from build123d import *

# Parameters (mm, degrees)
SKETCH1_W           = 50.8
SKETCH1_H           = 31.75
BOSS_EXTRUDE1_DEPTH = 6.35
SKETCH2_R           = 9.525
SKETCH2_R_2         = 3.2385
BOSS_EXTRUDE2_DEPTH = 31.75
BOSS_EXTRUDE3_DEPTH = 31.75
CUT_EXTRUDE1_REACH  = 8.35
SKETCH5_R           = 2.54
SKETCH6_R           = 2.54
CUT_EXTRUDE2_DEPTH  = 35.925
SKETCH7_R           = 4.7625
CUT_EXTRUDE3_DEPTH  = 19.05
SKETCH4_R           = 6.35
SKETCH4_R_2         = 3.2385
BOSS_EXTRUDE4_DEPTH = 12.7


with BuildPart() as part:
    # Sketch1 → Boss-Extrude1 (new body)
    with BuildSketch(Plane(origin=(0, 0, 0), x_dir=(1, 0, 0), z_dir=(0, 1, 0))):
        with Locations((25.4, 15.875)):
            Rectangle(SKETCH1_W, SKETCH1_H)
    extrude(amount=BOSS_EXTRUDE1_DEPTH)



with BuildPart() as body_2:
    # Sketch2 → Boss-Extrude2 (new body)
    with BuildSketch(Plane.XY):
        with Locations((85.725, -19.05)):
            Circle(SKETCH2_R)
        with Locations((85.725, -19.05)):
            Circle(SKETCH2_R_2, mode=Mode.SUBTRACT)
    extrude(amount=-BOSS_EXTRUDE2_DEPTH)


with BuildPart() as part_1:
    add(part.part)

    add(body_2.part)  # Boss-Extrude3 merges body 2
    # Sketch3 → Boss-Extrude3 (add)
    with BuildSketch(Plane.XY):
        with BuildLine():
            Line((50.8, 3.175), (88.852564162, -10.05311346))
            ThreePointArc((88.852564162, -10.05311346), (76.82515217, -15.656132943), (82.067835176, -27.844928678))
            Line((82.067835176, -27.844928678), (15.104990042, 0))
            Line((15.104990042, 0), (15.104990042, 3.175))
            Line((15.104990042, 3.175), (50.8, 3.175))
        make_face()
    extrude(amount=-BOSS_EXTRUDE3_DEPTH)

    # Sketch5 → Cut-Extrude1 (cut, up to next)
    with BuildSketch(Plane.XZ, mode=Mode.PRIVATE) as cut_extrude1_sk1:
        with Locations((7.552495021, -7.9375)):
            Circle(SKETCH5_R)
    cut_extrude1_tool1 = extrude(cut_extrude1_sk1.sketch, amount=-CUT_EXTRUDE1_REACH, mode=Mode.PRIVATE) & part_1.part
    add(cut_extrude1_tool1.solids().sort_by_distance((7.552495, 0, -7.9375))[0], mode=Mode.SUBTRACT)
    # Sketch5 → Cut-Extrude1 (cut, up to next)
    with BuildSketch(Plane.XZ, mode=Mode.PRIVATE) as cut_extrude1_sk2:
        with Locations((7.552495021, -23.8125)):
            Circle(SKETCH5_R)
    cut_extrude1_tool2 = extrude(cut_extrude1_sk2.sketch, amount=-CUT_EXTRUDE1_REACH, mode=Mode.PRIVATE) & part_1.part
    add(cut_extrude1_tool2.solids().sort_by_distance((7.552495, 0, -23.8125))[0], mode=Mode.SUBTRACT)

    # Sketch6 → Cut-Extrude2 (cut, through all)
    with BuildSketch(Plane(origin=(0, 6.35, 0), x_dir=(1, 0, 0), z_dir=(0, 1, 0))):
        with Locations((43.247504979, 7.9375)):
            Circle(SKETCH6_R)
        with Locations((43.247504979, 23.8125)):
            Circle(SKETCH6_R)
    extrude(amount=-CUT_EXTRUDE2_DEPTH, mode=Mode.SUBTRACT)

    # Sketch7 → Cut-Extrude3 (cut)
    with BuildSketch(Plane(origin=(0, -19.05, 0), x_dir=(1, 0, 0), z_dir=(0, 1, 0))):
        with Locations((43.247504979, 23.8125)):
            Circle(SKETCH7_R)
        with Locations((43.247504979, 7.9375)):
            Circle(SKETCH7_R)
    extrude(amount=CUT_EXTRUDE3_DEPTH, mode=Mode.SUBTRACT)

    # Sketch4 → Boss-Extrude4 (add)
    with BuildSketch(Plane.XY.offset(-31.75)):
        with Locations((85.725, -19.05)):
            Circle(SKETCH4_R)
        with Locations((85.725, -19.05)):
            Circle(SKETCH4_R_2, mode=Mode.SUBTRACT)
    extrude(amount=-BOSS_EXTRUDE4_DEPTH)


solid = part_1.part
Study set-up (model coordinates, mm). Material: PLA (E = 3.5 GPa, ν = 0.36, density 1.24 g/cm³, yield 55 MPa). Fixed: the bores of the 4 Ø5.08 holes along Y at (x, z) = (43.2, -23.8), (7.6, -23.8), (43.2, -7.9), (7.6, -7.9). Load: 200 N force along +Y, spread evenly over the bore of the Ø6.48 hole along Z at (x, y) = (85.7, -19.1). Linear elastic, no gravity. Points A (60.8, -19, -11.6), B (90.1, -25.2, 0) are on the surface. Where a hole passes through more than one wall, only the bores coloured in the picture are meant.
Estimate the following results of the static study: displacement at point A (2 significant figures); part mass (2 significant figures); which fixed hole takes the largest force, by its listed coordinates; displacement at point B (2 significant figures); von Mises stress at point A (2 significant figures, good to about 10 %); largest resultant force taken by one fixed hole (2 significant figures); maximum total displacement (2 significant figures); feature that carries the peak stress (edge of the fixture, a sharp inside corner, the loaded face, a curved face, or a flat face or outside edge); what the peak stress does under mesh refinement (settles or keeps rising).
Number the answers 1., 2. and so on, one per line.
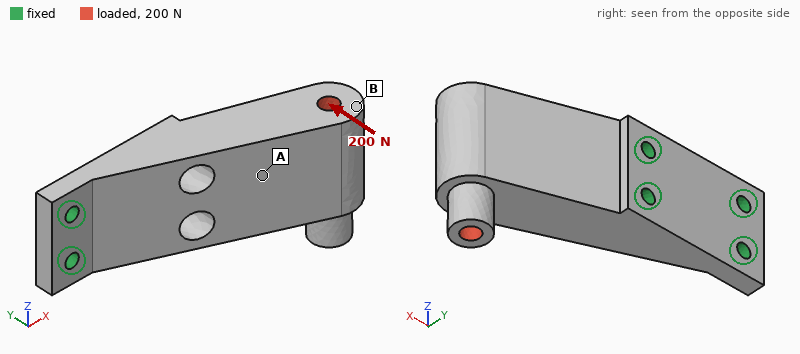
1. 0.14 mm
2. 53 g
3. (43.2, -23.8)
4. 0.32 mm
5. 2.6 MPa
6. 280 N
7. 0.39 mm
8. edge of the fixture
9. keeps rising
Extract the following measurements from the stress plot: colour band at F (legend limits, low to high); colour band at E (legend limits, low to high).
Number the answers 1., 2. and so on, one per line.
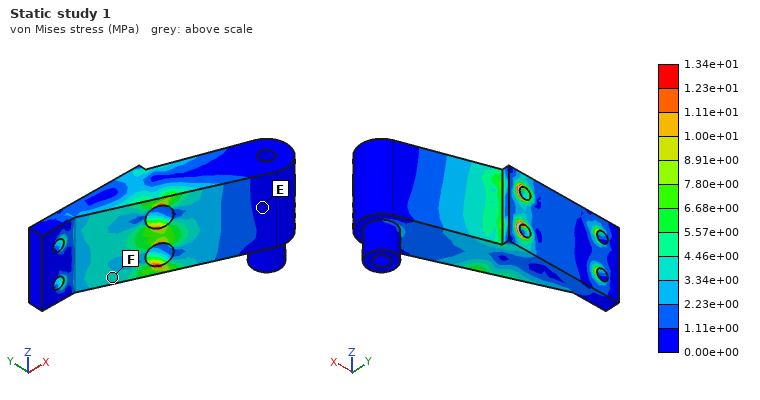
1. 3.34e+00 to 4.46e+00 MPa
2. 0.00e+00 to 1.11e+00 MPa
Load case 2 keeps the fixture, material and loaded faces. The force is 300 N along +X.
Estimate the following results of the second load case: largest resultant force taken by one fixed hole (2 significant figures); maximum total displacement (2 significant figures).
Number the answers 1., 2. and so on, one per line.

1. 130 N
2. 0.27 mm
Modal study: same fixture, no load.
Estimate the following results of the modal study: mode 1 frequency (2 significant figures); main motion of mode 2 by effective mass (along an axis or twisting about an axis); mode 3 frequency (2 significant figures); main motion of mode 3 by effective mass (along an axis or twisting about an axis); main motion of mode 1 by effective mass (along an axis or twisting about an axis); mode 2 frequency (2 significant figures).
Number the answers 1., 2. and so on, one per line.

1. 950 Hz
2. along Z
3. 2700 Hz
4. twisting about X
5. along Y
6. 1600 Hz
